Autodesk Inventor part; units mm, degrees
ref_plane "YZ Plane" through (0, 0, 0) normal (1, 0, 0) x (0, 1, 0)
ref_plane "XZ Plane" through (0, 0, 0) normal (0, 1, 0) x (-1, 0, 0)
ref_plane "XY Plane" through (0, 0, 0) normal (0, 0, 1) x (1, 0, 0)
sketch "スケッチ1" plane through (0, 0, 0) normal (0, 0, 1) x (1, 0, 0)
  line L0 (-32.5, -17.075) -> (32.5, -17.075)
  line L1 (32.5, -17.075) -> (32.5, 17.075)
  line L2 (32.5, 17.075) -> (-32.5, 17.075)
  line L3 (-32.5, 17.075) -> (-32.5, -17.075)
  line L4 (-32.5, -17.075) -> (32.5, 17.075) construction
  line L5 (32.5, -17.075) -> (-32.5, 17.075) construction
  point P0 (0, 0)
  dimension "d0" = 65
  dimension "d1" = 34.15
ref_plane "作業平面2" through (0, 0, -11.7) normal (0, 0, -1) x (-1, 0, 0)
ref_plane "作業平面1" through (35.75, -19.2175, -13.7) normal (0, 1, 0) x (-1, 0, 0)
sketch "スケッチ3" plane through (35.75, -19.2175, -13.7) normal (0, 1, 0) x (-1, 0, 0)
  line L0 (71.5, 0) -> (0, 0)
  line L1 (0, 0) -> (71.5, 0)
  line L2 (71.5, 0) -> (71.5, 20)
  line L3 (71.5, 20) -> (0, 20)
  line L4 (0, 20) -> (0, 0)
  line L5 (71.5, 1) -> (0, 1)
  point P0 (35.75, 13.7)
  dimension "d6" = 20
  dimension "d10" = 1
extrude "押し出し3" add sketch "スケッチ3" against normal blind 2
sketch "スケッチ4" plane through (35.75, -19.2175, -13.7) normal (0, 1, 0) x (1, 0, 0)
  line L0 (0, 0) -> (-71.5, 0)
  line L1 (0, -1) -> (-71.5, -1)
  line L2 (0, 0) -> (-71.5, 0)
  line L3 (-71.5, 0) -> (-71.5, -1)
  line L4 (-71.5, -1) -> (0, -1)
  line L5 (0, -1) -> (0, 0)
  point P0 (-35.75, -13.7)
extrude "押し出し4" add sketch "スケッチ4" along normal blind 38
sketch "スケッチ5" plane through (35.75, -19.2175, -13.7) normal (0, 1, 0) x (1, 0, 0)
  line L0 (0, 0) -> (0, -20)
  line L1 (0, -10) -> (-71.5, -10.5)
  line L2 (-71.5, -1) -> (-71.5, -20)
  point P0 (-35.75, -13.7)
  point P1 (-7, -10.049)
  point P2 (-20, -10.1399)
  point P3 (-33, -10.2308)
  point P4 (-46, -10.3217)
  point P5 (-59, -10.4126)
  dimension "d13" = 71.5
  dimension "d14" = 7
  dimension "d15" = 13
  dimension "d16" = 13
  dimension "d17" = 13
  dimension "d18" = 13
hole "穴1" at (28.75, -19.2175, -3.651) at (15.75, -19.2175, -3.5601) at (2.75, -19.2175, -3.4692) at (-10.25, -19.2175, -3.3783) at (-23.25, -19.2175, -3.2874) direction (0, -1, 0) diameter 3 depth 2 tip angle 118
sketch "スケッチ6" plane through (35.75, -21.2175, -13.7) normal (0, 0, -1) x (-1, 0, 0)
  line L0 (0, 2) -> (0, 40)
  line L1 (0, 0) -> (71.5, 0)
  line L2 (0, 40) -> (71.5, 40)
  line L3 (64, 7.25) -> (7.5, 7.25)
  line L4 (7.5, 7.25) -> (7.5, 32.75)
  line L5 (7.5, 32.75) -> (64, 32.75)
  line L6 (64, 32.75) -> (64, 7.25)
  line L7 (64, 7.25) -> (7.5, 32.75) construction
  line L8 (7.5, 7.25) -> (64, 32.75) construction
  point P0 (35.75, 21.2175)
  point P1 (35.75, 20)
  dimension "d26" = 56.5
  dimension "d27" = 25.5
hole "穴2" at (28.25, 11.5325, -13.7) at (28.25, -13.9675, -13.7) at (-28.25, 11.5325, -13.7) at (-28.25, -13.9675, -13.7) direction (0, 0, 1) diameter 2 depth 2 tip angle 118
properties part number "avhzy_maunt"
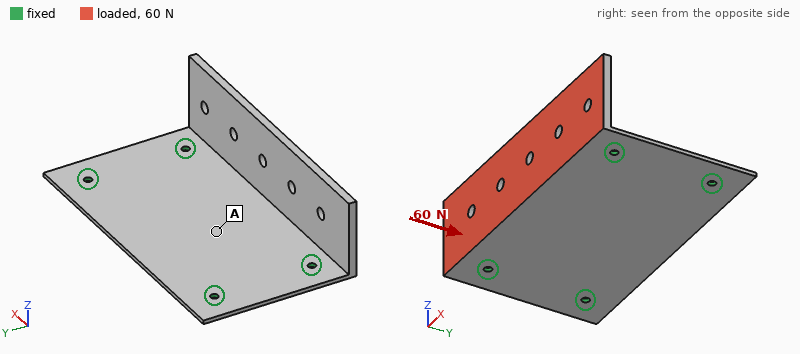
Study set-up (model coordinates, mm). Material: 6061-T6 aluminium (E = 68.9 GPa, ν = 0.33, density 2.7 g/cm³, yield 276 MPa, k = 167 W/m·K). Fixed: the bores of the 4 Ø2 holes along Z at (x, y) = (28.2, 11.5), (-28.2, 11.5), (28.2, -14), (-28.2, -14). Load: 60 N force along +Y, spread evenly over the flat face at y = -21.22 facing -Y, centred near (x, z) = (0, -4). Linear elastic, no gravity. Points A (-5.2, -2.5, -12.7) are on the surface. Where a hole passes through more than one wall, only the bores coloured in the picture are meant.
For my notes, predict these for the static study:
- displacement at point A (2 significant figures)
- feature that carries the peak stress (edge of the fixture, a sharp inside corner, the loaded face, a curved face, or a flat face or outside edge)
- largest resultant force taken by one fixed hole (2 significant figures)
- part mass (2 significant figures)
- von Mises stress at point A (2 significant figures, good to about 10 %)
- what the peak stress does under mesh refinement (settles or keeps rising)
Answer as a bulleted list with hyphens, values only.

- 0.046 mm
- edge of the fixture
- 21 N
- 15 g
- 11 MPa
- keeps rising
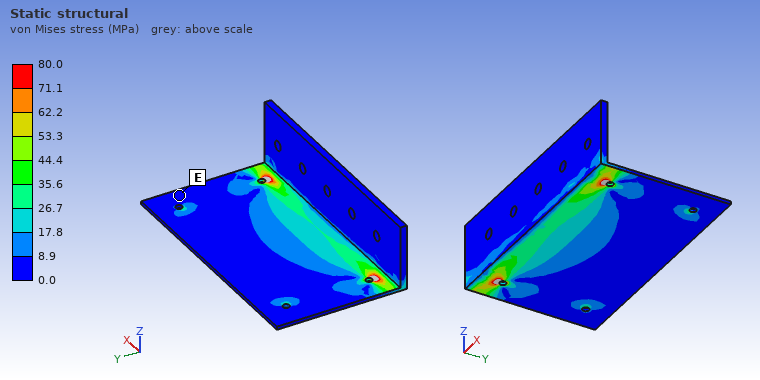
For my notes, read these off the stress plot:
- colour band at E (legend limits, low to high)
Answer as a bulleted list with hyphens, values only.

- 0.0 to 8.9 MPa
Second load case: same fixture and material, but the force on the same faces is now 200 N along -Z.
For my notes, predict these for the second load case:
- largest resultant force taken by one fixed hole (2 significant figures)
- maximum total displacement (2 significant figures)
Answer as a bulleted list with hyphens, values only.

- 120 N
- 0.37 mm
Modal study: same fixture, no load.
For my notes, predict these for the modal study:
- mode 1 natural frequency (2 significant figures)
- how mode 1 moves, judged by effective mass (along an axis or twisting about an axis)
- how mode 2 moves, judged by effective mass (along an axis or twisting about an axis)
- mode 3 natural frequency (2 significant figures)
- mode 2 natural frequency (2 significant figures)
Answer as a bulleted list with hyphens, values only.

- 1100 Hz
- along Y
- along Z
- 2400 Hz
- 1900 Hz
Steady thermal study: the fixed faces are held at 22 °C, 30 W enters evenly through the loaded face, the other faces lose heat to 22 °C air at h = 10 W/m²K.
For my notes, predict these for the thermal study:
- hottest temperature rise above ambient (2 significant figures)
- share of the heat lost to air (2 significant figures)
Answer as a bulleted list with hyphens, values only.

- 51 K
- 5.6 %
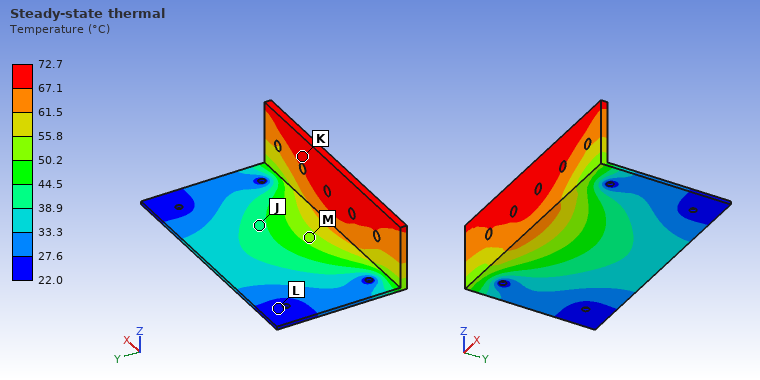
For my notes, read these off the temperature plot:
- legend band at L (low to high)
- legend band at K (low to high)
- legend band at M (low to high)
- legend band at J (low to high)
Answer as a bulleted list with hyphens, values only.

- 22.0 to 27.6 °C
- 67.1 to 72.7 °C
- 50.2 to 55.8 °C
- 38.9 to 44.5 °C
